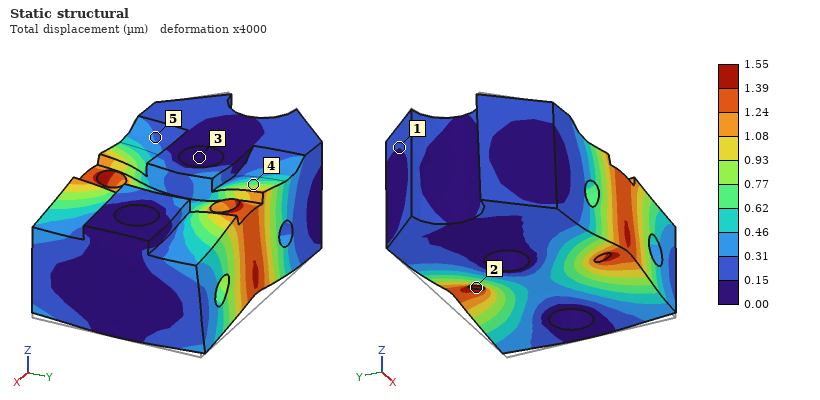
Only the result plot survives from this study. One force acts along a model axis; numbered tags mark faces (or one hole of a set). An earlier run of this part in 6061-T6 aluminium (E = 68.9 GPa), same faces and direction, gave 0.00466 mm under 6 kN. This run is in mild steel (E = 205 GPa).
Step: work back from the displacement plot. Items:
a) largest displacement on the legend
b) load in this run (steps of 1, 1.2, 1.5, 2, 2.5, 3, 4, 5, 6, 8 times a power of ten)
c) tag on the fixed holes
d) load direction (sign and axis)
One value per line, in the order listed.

1.55 µm
6 kN
3
+Z
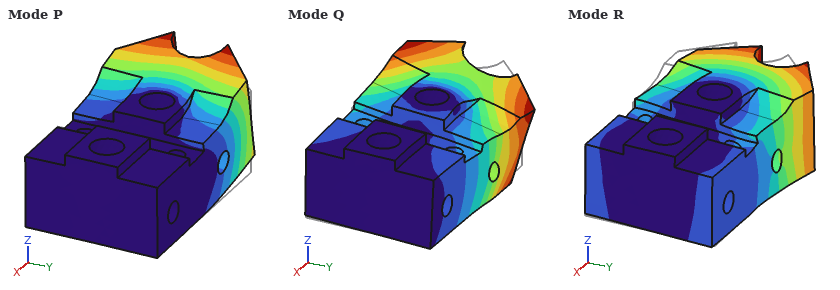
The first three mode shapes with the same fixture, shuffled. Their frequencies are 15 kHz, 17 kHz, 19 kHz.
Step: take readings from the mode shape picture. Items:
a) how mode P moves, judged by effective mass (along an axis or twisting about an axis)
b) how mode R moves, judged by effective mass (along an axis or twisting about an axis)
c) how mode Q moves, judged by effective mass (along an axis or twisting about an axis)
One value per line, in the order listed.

along Z
along Y
twisting about X
